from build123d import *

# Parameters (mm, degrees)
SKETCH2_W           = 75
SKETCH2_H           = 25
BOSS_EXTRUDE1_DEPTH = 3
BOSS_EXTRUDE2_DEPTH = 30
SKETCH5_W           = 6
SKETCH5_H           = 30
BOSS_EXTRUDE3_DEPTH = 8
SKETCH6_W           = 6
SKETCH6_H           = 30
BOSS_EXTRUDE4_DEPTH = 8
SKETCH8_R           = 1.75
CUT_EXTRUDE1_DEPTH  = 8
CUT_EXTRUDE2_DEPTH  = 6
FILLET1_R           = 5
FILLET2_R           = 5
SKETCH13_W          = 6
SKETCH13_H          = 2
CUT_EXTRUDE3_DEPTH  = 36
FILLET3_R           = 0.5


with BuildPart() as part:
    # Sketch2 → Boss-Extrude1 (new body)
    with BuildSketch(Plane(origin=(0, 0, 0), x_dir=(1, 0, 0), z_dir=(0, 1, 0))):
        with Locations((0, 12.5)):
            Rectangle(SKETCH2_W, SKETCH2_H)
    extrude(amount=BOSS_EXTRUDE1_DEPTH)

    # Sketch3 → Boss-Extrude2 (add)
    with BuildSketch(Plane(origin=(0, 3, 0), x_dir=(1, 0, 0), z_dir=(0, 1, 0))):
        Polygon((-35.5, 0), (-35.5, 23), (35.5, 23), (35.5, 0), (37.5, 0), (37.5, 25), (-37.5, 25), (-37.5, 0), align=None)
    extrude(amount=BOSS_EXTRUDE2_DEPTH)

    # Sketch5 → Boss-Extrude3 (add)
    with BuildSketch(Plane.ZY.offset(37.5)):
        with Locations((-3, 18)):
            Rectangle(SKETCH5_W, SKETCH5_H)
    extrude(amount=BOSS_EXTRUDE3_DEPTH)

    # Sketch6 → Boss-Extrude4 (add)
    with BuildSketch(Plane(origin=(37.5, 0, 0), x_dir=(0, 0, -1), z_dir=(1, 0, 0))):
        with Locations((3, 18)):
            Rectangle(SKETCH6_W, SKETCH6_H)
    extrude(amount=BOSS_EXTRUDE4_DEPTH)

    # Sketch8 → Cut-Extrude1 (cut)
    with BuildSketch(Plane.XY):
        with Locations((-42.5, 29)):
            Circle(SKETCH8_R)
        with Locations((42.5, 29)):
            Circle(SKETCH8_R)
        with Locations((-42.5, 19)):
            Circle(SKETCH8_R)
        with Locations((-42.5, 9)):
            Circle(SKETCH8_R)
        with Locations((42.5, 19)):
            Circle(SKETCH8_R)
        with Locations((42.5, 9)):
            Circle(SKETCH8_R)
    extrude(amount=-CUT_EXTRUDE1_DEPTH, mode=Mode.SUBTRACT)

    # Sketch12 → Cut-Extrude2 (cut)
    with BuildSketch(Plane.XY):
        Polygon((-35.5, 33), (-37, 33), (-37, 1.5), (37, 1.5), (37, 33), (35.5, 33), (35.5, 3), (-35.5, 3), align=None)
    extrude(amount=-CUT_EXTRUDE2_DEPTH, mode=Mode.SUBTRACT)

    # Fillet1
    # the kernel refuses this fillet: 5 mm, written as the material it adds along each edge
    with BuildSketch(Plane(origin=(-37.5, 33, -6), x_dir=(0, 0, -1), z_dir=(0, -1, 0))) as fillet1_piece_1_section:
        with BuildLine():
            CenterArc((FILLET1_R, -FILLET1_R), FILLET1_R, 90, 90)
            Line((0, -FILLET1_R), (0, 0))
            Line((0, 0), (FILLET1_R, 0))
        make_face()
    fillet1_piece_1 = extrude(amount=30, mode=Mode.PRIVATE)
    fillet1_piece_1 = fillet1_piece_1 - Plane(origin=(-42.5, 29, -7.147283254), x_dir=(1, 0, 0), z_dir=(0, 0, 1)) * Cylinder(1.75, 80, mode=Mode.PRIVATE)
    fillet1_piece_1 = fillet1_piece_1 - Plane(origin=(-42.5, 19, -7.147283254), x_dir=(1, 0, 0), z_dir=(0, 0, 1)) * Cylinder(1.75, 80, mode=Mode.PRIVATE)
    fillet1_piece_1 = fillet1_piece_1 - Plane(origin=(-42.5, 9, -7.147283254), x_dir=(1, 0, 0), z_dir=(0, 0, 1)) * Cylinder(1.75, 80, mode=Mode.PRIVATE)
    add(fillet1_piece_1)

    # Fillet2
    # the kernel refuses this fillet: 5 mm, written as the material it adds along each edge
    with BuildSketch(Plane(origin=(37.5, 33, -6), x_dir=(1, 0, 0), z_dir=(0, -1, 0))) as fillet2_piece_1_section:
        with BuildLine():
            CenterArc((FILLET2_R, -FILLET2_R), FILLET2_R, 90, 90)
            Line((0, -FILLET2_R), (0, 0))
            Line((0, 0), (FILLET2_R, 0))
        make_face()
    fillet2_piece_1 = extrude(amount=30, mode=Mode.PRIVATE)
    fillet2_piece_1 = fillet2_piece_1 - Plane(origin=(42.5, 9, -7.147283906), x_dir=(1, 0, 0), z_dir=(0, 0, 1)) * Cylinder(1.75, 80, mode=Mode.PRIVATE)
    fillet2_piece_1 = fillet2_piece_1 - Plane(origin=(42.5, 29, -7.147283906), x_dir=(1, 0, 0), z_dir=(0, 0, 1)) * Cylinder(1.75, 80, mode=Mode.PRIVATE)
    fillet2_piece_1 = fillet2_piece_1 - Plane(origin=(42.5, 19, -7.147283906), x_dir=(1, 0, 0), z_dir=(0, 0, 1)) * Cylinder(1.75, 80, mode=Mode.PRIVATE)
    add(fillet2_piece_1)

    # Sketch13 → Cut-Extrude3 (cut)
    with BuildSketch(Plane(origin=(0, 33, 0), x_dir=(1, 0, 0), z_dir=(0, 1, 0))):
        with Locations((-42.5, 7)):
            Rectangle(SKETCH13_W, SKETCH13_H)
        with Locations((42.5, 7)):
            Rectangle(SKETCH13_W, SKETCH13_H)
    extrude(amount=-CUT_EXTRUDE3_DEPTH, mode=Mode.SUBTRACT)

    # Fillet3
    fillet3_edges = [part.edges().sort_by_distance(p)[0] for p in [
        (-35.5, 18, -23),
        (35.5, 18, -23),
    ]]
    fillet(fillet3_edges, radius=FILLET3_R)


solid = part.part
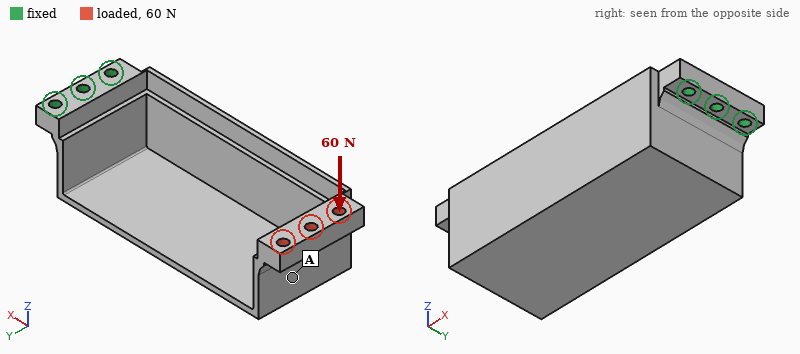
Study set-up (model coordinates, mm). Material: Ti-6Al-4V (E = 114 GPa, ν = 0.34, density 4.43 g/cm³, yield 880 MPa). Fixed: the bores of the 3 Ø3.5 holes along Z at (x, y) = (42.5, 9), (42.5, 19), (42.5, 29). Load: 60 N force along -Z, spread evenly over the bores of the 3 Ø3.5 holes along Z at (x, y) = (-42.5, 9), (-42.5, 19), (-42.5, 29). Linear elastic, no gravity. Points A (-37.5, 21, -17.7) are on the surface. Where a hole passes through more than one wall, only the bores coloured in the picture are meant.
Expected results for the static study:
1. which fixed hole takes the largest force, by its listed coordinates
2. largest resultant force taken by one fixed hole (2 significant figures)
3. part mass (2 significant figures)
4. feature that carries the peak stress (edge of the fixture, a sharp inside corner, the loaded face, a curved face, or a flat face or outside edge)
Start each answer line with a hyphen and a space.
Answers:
- (42.5, 19)
- 120 N
- 64 g
- a flat face or outside edge
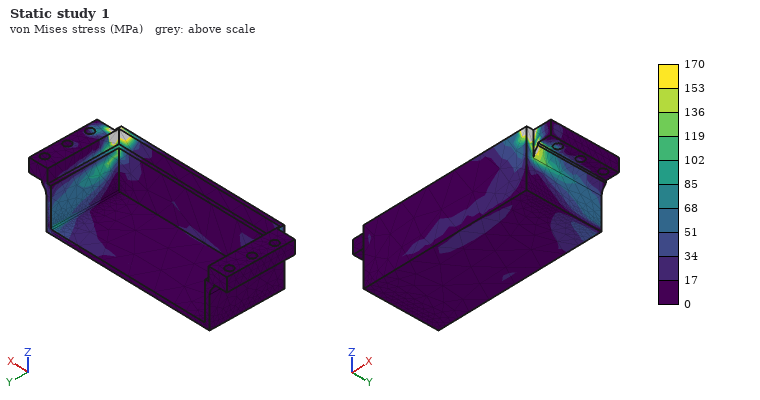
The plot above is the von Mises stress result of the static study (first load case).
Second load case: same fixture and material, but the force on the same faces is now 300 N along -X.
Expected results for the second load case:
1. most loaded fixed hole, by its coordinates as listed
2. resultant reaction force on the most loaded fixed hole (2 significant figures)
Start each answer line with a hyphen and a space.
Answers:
- (42.5, 29)
- 150 N
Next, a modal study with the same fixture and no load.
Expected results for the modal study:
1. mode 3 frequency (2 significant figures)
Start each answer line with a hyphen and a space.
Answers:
- 1200 Hz
